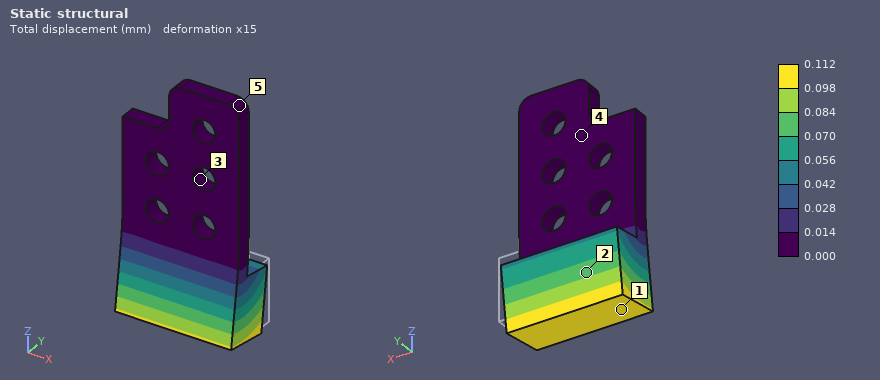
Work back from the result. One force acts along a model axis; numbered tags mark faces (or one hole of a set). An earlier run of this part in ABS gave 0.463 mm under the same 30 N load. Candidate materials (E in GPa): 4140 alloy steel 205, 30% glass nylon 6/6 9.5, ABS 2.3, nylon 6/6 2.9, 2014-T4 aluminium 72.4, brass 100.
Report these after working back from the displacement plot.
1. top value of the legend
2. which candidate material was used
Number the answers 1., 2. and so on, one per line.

1. 0.112 mm
2. 30% glass nylon 6/6
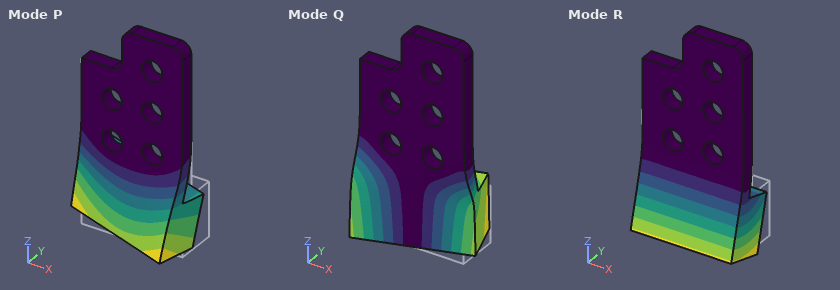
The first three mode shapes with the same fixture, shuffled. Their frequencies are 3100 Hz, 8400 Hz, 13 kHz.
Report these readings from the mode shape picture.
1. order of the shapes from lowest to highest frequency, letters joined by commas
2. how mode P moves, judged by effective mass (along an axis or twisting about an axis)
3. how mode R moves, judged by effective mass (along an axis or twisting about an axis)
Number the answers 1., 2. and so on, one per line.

1. R, Q, P
2. along X
3. along Y
